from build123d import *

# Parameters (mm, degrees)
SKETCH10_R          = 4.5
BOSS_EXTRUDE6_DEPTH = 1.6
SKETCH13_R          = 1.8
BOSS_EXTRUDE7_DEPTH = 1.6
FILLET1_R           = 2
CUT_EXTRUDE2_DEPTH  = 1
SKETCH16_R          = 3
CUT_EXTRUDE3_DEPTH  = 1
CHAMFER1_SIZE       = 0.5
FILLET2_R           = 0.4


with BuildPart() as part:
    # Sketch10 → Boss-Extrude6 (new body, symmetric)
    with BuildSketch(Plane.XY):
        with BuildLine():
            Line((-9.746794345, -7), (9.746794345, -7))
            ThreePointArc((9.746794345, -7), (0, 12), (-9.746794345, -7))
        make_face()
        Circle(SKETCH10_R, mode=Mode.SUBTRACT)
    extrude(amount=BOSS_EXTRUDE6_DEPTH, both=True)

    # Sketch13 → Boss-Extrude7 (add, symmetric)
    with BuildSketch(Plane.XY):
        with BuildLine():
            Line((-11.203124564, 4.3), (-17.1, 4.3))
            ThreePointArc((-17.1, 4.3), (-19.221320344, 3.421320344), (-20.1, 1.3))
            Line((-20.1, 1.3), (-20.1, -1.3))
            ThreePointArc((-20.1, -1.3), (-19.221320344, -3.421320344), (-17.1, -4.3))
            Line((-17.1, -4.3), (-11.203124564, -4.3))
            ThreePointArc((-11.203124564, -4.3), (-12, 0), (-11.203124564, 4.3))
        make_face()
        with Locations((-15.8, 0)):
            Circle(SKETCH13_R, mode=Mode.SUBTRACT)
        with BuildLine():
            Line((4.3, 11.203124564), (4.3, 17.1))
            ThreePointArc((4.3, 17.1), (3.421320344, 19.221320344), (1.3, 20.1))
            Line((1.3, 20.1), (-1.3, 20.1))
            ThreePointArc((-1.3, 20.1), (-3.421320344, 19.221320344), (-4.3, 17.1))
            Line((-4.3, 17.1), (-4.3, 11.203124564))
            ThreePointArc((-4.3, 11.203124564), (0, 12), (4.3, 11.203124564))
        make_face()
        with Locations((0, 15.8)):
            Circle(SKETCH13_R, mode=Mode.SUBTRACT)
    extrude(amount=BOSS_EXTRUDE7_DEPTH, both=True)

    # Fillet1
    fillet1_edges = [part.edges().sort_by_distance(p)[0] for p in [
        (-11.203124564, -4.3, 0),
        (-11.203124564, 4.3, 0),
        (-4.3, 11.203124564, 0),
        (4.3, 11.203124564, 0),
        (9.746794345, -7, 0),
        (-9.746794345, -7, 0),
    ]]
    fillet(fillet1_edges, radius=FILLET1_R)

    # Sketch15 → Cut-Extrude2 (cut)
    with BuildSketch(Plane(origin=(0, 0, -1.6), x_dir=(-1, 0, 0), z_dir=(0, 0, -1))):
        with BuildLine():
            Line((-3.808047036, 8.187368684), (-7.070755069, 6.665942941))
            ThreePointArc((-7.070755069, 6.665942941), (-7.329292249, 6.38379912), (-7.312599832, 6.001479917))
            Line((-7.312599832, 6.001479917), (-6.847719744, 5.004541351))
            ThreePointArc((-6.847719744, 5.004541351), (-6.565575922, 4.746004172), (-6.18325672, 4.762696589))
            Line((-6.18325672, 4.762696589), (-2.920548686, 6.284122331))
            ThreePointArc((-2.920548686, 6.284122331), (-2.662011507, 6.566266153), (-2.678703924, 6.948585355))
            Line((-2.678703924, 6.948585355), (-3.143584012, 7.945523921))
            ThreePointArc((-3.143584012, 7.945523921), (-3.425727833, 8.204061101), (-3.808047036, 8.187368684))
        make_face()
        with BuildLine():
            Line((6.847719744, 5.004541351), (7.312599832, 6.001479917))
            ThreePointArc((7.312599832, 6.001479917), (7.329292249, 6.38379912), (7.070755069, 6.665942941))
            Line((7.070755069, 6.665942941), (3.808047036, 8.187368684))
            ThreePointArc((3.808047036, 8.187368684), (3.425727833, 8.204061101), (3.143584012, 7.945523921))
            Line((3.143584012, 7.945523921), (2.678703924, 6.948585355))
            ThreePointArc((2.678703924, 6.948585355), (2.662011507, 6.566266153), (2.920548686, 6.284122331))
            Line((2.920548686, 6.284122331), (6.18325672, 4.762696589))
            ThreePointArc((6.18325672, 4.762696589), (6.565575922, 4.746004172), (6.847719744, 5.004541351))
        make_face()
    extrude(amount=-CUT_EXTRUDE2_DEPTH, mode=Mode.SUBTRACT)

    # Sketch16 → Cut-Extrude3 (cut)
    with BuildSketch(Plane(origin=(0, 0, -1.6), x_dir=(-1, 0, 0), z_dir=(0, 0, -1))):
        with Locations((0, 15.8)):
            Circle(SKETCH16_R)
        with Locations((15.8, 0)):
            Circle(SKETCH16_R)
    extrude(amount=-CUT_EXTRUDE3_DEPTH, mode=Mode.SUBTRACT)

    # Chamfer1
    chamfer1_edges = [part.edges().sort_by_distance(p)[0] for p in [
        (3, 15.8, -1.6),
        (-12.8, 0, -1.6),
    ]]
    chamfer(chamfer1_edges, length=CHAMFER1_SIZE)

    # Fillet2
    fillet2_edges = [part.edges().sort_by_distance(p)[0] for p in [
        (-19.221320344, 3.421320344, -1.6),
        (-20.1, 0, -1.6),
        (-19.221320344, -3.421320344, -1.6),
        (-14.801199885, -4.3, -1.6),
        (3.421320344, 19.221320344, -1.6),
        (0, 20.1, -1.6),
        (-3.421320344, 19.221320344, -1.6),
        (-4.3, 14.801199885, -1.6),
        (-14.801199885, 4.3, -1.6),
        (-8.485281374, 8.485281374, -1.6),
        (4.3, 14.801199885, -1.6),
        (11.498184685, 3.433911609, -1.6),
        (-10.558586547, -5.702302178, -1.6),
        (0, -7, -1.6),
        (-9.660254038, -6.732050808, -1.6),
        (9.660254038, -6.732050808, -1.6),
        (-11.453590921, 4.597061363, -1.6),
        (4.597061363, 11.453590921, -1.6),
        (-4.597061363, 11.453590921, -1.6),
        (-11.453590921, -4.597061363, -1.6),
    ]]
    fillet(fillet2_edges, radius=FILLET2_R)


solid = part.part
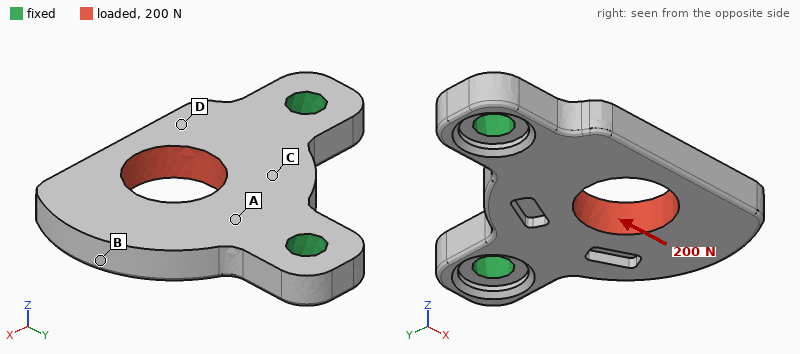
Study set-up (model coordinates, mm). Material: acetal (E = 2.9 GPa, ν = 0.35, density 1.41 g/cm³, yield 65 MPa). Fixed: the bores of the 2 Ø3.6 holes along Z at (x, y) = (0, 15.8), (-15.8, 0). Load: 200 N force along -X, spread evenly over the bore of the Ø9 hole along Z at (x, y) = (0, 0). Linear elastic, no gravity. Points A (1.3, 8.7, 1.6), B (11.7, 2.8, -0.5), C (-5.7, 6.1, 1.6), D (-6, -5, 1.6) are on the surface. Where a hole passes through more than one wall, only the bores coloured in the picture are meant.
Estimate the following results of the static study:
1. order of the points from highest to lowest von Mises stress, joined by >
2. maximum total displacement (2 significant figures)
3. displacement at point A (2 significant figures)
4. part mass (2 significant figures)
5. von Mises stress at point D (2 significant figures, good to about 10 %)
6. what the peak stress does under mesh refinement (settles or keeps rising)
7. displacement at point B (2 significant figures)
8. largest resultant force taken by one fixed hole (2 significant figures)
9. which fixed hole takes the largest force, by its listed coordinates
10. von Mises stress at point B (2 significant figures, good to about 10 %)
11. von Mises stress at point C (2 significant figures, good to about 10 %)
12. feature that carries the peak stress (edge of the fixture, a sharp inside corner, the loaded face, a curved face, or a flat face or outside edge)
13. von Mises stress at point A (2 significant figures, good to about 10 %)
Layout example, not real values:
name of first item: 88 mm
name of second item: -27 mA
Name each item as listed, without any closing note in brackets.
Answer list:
order of the points from highest to lowest von Mises stress, joined by >: D > C > B > A
maximum total displacement: 79 µm
displacement at point A: 21 µm
part mass: 1.9 g
von Mises stress at point D: 6.9 MPa
what the peak stress does under mesh refinement: keeps rising
displacement at point B: 64 µm
largest resultant force taken by one fixed hole: 170 N
which fixed hole takes the largest force, by its listed coordinates: (-15.8, 0)
von Mises stress at point B: 2.6 MPa
von Mises stress at point C: 4.6 MPa
feature that carries the peak stress: edge of the fixture
von Mises stress at point A: 1.2 MPa
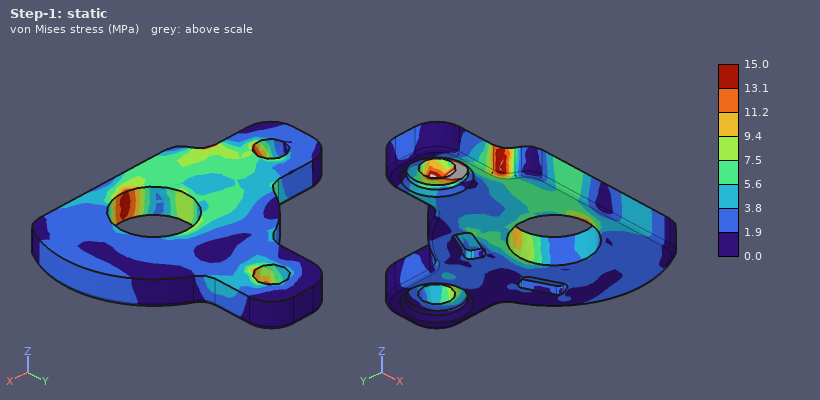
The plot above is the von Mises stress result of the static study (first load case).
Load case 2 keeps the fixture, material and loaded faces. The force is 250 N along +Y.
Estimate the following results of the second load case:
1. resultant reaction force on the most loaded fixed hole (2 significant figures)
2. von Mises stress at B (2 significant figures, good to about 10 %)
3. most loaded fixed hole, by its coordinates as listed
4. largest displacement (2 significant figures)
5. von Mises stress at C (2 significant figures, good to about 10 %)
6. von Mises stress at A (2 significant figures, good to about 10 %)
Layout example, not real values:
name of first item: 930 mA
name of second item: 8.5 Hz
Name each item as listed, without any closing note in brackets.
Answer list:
resultant reaction force on the most loaded fixed hole: 210 N
von Mises stress at B: 2.9 MPa
most loaded fixed hole, by its coordinates as listed: (0, 15.8)
largest displacement: 0.11 mm
von Mises stress at C: 6.4 MPa
von Mises stress at A: 7.2 MPa
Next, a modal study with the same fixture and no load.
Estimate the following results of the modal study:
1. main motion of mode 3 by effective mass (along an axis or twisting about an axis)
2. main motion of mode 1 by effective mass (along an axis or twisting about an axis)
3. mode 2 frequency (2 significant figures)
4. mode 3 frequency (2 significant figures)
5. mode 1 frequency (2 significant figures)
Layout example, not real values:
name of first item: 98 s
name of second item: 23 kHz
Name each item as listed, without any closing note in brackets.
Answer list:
main motion of mode 3 by effective mass: along Z
main motion of mode 1 by effective mass: along Z
mode 2 frequency: 4900 Hz
mode 3 frequency: 7100 Hz
mode 1 frequency: 1500 Hz
